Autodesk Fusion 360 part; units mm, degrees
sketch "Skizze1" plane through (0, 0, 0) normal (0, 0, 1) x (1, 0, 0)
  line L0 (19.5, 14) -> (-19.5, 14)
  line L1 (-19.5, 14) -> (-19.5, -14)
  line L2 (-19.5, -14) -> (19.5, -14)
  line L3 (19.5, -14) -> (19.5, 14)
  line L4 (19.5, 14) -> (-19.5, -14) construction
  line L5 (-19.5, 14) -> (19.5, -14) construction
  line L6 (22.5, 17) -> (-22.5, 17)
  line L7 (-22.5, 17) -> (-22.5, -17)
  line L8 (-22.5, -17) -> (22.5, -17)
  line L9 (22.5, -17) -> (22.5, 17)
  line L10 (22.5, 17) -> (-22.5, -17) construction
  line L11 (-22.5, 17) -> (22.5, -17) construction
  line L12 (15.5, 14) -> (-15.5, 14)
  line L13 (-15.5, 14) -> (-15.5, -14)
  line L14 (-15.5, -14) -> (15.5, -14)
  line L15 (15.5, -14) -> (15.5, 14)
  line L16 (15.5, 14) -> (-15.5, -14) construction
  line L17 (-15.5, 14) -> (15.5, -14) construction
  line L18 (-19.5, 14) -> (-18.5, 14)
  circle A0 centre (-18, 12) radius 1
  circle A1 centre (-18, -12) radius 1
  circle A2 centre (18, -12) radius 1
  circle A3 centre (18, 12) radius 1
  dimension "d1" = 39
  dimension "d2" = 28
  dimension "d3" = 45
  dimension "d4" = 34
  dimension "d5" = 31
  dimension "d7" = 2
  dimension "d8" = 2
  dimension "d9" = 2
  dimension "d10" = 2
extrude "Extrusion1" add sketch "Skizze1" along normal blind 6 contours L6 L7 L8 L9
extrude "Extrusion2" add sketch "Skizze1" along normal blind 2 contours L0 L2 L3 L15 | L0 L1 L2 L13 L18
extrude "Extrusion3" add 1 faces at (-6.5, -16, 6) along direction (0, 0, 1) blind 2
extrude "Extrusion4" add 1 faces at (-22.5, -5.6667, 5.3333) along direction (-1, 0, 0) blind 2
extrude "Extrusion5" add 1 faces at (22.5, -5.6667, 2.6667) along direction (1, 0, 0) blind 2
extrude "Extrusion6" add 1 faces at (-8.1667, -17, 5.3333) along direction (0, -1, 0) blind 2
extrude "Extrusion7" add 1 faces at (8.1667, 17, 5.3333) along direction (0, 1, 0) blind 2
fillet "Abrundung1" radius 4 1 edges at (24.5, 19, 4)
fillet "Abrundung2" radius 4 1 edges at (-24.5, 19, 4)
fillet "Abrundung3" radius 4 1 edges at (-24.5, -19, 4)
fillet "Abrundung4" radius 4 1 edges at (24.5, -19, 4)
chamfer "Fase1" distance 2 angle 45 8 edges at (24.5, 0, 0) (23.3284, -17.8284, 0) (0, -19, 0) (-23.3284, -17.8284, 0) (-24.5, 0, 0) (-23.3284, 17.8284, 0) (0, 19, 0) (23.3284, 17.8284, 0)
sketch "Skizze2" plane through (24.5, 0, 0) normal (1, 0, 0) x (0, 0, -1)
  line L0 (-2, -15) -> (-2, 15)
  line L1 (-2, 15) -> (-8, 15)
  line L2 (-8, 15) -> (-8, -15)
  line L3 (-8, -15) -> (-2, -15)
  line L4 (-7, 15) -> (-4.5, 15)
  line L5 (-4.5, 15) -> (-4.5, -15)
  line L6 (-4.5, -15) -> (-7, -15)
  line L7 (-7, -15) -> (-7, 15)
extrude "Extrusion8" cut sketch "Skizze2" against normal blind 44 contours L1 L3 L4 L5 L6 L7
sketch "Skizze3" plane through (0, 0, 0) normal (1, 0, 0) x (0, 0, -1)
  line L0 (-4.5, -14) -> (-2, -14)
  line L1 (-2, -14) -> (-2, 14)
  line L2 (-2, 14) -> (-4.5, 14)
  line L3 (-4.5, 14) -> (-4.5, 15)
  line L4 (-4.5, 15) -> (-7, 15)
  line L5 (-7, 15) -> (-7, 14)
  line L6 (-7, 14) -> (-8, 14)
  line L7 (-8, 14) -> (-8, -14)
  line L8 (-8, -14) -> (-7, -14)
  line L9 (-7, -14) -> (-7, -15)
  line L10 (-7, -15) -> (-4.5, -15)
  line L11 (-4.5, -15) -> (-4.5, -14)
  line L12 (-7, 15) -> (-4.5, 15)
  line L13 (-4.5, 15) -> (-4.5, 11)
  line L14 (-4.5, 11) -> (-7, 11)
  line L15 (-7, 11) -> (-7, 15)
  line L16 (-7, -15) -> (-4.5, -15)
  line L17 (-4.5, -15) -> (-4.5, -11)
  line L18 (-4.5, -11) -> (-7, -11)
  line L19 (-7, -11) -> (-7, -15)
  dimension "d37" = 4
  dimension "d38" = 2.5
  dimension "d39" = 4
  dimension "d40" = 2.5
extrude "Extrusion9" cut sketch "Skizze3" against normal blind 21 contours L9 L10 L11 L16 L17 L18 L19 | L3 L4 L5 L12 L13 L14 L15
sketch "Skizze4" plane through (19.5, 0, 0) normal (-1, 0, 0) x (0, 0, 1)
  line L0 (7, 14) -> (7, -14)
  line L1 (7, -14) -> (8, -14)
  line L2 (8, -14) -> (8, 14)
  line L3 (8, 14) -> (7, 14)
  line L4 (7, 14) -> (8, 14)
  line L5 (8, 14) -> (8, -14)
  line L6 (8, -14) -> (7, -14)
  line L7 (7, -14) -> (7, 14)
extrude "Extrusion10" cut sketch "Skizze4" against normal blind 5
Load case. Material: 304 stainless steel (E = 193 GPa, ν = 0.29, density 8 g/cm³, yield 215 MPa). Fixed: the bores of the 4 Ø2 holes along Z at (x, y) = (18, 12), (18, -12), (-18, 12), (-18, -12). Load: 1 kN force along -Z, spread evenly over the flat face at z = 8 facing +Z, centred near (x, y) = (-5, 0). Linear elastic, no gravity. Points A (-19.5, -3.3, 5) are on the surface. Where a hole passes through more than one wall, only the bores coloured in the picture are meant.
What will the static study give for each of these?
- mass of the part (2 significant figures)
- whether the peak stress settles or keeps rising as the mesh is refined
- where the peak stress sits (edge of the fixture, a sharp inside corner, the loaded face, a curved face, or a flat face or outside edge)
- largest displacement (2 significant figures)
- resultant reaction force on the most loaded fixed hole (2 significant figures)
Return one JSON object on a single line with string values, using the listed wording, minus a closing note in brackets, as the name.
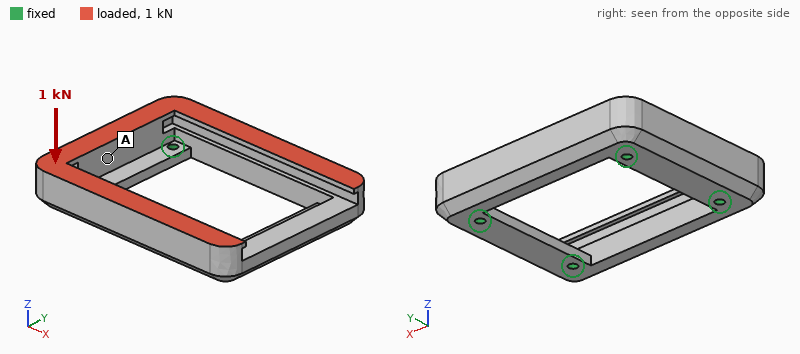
{"mass of the part": "43 g", "whether the peak stress settles or keeps rising as the mesh is refined": "keeps rising", "where the peak stress sits": "edge of the fixture", "largest displacement": "7.9 µm", "resultant reaction force on the most loaded fixed hole": "320 N"}
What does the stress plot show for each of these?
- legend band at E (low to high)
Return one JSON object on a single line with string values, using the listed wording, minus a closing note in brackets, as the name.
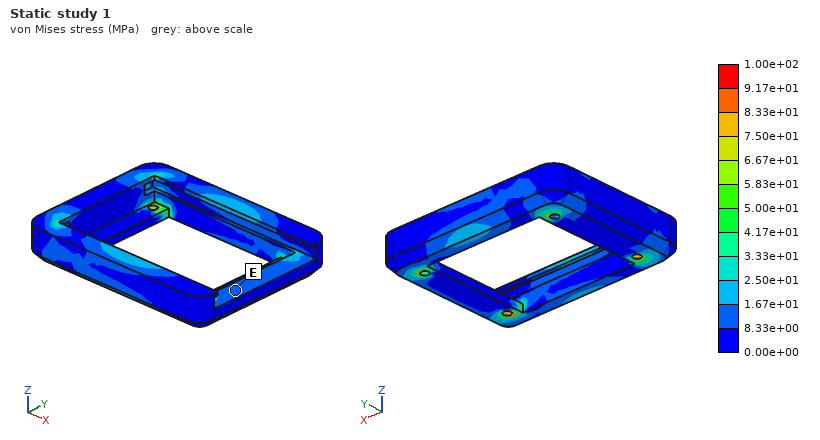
{"legend band at E": "8.33e+00 to 1.67e+01 MPa"}
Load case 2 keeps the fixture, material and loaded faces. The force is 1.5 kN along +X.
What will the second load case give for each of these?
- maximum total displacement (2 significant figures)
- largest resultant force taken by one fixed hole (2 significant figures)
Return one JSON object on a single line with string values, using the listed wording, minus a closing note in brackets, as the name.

{"maximum total displacement": "9.9 µm", "largest resultant force taken by one fixed hole": "440 N"}
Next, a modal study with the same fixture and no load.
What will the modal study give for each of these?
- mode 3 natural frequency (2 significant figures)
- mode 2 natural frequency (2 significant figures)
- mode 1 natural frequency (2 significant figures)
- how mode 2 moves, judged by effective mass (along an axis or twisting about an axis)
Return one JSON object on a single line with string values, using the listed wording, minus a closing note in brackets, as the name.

{"mode 3 natural frequency": "16 kHz", "mode 2 natural frequency": "10 kHz", "mode 1 natural frequency": "9000 Hz", "how mode 2 moves, judged by effective mass": "along Y"}
